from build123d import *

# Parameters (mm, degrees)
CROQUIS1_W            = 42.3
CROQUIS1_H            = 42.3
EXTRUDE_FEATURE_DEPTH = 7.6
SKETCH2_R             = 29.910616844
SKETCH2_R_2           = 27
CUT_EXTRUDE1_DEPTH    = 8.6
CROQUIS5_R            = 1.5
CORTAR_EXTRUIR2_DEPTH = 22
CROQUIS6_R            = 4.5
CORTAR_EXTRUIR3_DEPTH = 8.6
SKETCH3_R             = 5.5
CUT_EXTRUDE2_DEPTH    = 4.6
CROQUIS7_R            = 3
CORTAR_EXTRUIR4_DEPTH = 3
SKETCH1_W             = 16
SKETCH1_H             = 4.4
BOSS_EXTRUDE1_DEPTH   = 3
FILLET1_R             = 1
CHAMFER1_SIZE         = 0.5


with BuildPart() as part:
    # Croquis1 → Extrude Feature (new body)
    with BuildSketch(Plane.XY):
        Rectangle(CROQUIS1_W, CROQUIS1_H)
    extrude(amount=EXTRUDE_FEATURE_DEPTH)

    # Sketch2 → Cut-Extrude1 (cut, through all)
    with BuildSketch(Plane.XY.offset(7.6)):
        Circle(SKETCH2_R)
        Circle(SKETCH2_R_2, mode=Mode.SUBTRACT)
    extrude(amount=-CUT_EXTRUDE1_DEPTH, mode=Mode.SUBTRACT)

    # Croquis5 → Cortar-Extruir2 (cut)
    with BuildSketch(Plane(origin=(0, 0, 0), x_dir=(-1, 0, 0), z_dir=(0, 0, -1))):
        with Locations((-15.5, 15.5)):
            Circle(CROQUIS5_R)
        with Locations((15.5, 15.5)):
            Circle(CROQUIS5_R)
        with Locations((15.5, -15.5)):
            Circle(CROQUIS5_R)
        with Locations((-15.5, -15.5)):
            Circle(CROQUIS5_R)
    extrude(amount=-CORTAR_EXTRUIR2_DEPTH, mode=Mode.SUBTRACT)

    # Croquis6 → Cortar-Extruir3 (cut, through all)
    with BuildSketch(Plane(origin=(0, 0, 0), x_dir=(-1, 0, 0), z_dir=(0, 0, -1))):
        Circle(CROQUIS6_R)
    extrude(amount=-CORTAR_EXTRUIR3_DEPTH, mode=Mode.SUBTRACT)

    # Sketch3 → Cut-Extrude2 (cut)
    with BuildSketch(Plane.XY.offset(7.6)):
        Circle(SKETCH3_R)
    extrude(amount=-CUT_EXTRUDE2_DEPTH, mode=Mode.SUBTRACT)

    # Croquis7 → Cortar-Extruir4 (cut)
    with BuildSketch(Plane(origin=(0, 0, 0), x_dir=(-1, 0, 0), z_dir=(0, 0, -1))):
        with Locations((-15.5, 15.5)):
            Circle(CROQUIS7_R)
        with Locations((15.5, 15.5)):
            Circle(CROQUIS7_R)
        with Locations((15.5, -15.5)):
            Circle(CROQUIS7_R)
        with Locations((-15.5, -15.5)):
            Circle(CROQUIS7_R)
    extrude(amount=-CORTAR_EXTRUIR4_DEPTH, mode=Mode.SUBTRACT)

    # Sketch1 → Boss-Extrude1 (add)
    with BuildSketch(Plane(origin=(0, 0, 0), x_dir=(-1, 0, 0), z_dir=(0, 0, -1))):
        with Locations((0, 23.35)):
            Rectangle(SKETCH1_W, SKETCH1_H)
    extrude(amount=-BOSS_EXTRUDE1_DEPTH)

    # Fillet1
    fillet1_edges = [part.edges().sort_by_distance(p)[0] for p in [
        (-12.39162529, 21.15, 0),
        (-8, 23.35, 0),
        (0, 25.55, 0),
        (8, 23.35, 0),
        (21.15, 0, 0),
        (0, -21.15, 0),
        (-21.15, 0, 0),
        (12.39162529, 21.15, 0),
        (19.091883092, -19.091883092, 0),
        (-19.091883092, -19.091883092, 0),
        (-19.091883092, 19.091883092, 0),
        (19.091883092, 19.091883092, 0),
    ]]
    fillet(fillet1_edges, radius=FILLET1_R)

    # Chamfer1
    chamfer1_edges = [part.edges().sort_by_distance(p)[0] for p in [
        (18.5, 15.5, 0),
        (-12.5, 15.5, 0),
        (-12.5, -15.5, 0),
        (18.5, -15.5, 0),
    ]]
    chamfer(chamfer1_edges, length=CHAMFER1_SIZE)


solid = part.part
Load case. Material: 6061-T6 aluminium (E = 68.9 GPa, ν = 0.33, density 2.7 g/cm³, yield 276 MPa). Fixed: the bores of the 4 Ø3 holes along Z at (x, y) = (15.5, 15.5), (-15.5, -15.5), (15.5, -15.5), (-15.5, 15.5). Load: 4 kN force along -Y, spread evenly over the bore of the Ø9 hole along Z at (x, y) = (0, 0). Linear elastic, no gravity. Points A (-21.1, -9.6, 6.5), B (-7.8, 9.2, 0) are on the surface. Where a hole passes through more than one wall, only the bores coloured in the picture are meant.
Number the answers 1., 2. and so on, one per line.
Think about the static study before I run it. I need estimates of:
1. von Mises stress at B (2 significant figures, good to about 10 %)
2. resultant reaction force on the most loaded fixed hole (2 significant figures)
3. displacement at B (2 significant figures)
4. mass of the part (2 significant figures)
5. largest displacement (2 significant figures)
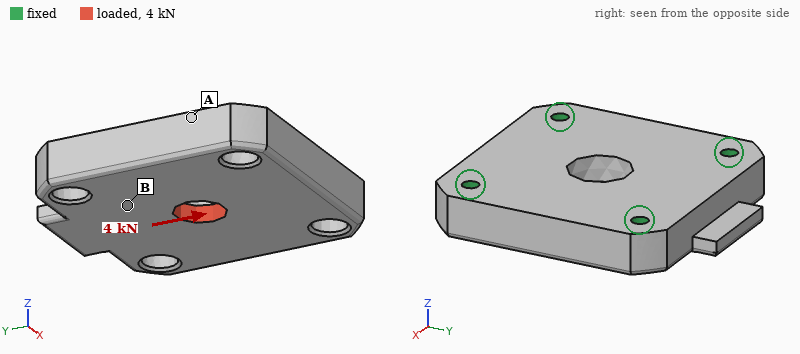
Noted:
1. 21 MPa
2. 1.1 kN
3. 3.9 µm
4. 33 g
5. 9.0 µm
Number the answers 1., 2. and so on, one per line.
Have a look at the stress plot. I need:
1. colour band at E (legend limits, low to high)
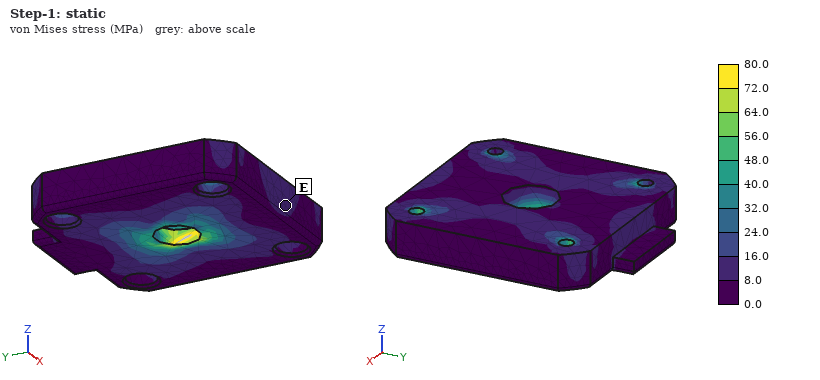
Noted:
1. 8.0 to 16.0 MPa
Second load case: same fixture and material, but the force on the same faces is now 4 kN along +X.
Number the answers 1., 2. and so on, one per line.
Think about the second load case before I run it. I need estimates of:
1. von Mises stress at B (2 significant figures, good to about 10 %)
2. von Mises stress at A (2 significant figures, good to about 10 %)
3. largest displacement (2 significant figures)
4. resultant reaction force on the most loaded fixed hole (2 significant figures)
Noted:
1. 19 MPa
2. 5.2 MPa
3. 9.1 µm
4. 1.1 kN
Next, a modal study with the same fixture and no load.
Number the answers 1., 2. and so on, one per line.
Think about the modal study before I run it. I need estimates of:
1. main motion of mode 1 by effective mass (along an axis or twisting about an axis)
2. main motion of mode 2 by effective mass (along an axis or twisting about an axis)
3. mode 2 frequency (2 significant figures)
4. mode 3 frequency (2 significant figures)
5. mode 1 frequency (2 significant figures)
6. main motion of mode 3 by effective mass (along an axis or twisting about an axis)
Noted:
1. along Z
2. twisting about X
3. 24 kHz
4. 27 kHz
5. 19 kHz
6. twisting about X
